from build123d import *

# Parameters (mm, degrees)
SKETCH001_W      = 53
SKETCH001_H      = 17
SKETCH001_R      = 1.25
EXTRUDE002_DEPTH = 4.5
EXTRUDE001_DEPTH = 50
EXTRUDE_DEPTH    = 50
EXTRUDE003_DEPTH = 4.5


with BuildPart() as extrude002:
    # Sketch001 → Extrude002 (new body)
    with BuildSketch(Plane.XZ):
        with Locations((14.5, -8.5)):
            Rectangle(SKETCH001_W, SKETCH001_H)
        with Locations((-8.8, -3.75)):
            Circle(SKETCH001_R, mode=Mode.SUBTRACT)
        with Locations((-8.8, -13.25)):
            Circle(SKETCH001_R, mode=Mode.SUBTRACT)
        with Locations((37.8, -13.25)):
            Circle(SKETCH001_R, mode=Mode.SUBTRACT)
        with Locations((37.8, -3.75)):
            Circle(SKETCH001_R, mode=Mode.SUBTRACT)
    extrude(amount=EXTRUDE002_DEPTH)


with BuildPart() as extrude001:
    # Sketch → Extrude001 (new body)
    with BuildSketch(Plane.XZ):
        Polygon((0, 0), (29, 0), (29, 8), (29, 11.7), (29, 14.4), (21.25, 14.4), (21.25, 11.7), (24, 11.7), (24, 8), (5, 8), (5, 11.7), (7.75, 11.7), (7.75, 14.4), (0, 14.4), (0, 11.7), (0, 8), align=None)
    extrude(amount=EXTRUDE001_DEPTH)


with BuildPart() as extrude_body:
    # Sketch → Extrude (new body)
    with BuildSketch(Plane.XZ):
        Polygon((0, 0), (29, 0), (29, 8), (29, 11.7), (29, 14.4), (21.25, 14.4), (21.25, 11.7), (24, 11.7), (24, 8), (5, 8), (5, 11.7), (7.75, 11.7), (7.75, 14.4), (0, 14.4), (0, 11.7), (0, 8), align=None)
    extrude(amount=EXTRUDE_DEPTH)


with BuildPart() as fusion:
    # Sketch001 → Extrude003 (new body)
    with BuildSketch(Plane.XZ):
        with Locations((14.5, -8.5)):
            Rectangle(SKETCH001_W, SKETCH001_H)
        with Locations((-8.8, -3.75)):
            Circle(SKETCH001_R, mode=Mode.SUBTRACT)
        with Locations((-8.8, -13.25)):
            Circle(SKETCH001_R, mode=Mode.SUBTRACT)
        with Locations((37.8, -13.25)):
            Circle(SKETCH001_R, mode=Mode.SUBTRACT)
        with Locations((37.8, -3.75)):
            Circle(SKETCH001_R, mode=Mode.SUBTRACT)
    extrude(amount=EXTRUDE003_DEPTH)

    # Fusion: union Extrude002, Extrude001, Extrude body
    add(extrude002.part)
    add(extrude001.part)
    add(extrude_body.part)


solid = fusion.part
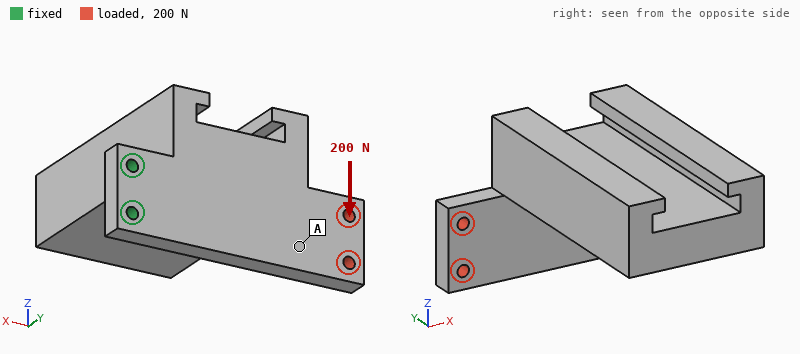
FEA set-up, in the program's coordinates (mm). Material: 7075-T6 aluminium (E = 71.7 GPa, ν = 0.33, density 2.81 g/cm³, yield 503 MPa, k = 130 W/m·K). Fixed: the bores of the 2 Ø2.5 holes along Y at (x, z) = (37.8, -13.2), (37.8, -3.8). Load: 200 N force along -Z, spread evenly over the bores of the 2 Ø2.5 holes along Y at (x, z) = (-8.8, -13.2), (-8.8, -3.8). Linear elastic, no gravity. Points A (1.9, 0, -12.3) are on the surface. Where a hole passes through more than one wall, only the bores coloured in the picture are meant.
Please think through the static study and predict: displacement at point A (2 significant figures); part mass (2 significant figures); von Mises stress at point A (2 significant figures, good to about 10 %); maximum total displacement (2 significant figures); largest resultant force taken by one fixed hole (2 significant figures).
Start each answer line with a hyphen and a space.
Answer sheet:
- 35 µm
- 55 g
- 4.3 MPa
- 54 µm
- 850 N
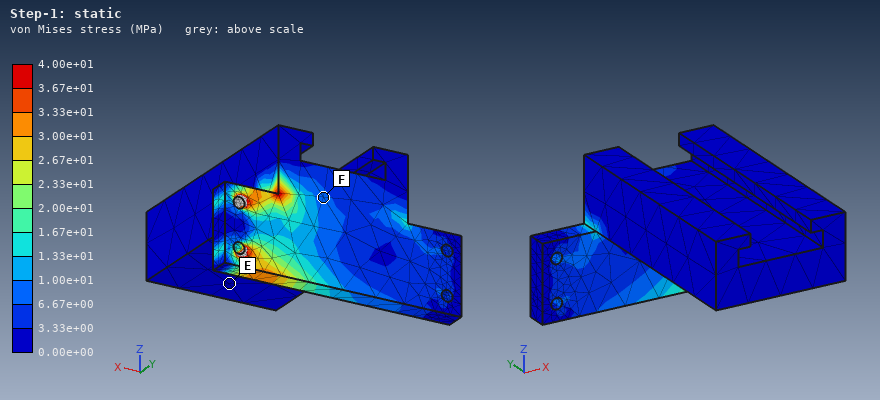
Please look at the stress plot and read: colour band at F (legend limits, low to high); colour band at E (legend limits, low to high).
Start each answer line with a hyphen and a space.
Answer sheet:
- 6.67e+00 to 1.00e+01 MPa
- 0.00e+00 to 3.33e+00 MPa
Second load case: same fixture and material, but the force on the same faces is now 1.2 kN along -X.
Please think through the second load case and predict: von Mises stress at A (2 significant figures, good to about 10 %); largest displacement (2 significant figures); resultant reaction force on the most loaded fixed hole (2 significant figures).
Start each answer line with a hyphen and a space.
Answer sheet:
- 16 MPa
- 14 µm
- 600 N
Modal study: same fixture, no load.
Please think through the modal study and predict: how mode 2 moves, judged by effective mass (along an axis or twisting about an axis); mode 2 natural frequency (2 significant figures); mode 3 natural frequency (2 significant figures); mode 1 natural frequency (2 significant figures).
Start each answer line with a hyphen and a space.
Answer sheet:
- along Z
- 730 Hz
- 3100 Hz
- 520 Hz
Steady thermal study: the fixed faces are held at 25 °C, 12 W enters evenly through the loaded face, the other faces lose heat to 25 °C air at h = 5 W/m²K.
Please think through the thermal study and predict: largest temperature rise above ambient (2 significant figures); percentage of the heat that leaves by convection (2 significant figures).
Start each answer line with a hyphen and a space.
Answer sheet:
- 46 K
- 7.2 %
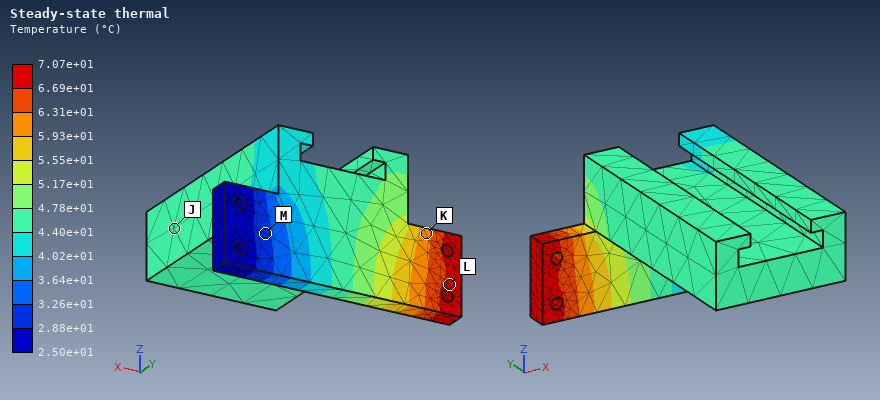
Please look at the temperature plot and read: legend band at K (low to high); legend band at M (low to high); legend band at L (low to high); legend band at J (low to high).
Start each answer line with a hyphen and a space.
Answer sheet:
- 5.93e+01 to 6.31e+01 °C
- 2.88e+01 to 3.26e+01 °C
- 6.69e+01 to 7.07e+01 °C
- 4.40e+01 to 4.78e+01 °C
